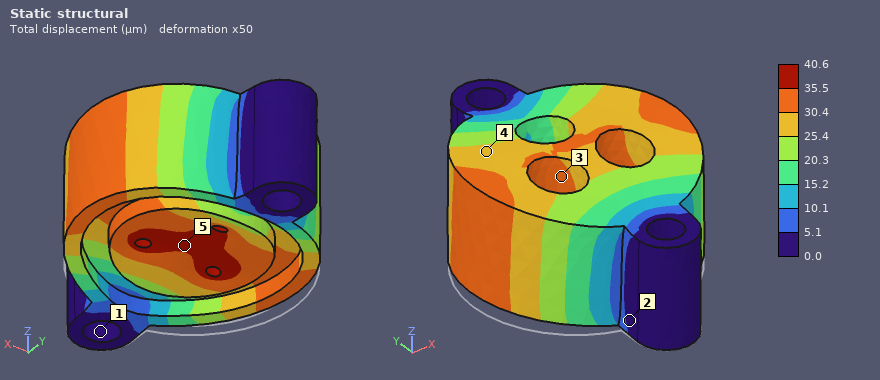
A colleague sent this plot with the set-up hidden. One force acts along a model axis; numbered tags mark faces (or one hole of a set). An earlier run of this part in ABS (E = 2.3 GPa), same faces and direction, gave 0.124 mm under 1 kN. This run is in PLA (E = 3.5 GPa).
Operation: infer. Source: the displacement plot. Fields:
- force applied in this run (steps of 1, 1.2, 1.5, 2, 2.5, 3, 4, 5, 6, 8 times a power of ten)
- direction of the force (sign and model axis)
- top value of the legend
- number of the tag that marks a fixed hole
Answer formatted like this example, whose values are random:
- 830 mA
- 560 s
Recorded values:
- 500 N
- +Z
- 40.6 µm
- 1
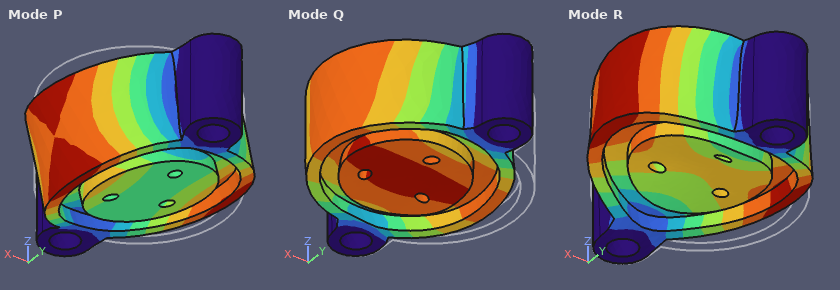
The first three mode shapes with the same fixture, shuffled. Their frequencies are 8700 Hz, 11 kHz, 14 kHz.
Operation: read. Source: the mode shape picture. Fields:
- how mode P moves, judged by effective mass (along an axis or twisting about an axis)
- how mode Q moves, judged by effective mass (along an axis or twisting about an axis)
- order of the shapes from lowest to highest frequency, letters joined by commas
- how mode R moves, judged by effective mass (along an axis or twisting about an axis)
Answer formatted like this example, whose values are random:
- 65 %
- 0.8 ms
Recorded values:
- twisting about Y
- along X
- P, R, Q
- along Z
